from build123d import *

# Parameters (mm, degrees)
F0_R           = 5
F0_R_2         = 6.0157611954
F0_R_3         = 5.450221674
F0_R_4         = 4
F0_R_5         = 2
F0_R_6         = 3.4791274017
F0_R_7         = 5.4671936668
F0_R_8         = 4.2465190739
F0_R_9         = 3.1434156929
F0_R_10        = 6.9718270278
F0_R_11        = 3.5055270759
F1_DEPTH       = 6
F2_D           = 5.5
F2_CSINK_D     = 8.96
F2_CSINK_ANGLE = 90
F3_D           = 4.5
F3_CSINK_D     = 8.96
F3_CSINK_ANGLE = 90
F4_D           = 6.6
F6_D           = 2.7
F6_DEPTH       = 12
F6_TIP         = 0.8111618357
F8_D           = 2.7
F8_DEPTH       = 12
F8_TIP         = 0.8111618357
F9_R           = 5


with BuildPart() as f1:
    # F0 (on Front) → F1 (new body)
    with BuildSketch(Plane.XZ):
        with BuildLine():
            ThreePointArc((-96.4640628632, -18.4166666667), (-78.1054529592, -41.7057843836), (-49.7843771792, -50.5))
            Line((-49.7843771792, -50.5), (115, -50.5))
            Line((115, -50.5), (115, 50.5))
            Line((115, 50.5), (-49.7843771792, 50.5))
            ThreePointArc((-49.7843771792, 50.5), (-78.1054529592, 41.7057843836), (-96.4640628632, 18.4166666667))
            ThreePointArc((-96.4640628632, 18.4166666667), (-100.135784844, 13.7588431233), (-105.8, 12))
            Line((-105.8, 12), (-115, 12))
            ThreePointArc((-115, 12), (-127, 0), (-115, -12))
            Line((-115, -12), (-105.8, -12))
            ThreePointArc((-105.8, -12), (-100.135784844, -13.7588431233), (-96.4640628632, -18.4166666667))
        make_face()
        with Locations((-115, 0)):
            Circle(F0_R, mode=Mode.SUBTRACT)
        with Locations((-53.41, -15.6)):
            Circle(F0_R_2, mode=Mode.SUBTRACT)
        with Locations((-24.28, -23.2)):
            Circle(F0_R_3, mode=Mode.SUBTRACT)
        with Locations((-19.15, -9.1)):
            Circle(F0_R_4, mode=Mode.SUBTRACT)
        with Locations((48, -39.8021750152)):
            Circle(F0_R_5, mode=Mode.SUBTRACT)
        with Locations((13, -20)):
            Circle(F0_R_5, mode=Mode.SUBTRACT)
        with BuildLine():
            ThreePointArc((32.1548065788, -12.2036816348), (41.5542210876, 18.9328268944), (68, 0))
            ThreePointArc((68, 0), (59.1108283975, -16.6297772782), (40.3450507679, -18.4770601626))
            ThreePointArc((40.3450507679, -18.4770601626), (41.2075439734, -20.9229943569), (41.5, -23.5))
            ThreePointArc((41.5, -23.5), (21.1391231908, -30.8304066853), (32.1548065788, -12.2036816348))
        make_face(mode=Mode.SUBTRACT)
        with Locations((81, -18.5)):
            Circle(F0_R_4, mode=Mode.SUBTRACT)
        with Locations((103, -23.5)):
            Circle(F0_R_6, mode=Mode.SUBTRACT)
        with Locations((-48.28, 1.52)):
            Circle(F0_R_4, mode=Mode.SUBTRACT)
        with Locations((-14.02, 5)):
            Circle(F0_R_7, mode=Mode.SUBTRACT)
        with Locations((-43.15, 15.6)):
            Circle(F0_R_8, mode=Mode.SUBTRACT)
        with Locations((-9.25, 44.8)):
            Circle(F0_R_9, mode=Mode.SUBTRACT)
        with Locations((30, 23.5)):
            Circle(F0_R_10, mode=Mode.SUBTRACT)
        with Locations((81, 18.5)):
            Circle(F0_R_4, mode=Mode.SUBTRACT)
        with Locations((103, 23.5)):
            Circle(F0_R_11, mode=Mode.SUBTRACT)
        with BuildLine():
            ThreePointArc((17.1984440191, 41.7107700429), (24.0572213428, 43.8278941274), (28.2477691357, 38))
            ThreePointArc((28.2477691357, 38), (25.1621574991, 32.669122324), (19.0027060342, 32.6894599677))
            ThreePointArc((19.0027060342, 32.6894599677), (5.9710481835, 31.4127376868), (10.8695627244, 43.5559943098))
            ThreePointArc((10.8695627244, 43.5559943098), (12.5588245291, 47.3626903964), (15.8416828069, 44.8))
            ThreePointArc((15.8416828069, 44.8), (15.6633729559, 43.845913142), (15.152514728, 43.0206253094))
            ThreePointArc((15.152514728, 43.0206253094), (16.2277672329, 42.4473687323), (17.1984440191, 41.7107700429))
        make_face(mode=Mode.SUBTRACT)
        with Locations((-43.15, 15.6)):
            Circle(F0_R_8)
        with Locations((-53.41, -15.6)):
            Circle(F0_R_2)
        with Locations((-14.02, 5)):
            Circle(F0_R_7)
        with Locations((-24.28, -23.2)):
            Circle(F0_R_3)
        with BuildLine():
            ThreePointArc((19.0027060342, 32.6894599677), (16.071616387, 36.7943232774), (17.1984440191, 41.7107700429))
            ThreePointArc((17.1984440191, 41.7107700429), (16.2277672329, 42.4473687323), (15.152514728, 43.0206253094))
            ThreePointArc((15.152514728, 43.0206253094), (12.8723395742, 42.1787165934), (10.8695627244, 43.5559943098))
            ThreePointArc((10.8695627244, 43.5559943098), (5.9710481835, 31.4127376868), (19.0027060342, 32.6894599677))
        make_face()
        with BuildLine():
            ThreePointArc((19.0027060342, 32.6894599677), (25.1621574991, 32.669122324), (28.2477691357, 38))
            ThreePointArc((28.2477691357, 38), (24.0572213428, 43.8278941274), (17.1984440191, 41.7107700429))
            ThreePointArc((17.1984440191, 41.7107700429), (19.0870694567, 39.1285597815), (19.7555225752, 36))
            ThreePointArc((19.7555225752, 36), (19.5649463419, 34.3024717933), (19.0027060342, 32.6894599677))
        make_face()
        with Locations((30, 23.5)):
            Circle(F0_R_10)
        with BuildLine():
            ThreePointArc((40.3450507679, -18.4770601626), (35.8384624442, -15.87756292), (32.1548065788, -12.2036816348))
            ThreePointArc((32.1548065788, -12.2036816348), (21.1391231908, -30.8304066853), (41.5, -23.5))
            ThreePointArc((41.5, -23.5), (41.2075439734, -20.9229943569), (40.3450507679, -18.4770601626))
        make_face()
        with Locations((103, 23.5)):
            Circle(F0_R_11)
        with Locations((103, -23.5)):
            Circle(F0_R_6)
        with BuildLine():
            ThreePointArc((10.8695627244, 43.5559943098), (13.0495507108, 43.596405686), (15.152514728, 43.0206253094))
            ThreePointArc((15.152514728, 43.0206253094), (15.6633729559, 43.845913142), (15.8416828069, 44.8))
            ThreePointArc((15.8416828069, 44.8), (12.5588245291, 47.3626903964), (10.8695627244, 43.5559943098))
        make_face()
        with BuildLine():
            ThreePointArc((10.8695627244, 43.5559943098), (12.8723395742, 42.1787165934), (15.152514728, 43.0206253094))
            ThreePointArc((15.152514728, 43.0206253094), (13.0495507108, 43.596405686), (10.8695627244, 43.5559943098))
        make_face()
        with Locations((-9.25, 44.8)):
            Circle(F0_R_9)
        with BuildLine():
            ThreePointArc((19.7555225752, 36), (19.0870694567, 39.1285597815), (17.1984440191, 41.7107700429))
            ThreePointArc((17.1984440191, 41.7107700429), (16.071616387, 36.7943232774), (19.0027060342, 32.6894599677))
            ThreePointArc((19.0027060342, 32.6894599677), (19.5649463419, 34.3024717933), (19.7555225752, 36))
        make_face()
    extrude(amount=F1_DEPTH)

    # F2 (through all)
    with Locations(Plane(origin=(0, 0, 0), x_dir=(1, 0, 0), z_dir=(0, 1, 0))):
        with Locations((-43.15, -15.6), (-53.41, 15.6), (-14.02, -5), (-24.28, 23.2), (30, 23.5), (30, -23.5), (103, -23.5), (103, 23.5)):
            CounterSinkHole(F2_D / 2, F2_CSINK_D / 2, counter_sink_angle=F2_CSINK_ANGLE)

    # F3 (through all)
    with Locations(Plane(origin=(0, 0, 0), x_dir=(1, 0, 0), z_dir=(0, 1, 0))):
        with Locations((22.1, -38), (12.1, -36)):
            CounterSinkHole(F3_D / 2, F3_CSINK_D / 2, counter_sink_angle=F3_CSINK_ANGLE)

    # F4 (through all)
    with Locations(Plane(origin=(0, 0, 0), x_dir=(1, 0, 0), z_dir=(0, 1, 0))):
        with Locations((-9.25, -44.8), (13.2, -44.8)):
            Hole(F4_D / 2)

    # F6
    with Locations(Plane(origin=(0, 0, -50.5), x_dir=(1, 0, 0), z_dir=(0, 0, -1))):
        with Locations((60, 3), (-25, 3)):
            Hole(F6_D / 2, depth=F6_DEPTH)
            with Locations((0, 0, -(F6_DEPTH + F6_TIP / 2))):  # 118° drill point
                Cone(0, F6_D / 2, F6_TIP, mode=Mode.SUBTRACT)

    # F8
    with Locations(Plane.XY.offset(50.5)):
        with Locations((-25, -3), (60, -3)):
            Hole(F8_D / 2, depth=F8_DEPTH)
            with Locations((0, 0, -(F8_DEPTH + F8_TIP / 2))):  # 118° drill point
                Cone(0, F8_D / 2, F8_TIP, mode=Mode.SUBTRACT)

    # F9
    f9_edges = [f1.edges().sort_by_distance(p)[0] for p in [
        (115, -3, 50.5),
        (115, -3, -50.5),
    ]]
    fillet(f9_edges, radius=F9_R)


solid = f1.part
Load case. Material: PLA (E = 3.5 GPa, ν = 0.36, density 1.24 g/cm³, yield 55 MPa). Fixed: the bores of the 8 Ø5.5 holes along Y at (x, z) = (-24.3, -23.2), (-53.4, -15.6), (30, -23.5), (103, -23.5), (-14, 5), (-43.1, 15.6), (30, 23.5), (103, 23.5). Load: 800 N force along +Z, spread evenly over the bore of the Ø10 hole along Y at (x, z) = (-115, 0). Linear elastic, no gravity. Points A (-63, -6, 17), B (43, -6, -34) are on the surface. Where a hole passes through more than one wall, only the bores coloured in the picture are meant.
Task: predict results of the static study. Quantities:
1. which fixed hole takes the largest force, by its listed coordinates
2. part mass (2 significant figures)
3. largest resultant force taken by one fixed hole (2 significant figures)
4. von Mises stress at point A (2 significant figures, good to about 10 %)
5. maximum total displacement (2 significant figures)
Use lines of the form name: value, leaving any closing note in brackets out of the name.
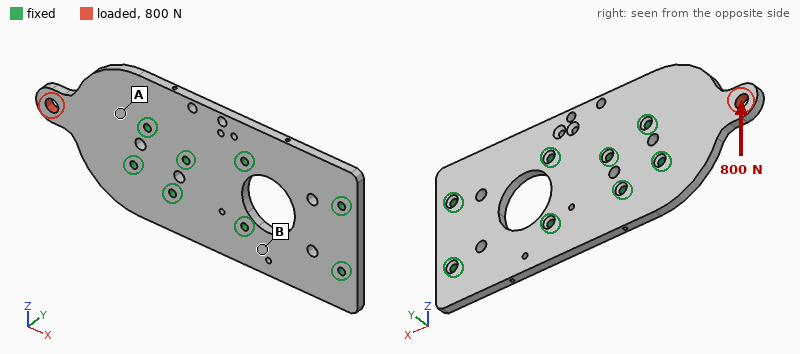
which fixed hole takes the largest force, by its listed coordinates: (-53.4, -15.6)
part mass: 140 g
largest resultant force taken by one fixed hole: 860 N
von Mises stress at point A: 4.8 MPa
maximum total displacement: 0.55 mm
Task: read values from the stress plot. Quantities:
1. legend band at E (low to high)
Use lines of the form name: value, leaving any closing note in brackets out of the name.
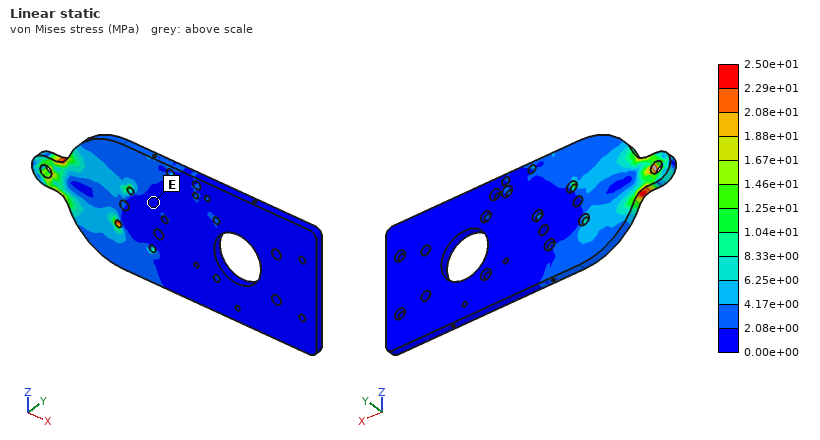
legend band at E: 0.00e+00 to 2.08e+00 MPa
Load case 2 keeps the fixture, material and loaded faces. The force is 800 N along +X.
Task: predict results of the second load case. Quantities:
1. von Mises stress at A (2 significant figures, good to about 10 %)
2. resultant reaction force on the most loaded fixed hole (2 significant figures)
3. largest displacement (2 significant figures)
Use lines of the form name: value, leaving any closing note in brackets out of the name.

von Mises stress at A: 2.2 MPa
resultant reaction force on the most loaded fixed hole: 310 N
largest displacement: 0.10 mm
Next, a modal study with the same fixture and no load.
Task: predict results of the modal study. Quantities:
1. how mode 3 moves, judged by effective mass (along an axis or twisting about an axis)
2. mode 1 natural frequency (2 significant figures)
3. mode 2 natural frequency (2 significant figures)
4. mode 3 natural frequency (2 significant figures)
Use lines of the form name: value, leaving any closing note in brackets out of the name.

how mode 3 moves, judged by effective mass: along Y
mode 1 natural frequency: 460 Hz
mode 2 natural frequency: 1000 Hz
mode 3 natural frequency: 1300 Hz
